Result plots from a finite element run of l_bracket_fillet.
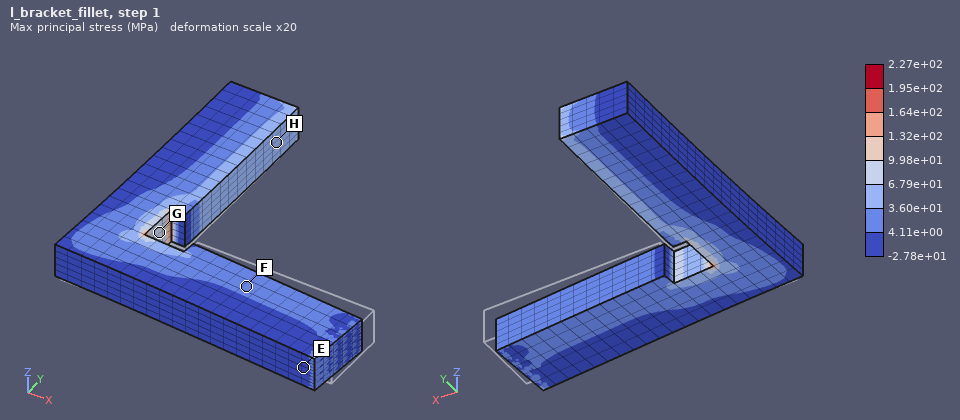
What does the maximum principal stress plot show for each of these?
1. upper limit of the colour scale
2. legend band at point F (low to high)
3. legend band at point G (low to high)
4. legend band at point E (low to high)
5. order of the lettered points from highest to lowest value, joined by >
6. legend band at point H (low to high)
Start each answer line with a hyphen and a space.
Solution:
- 2.27e+02 MPa
- 4.11e+00 to 3.60e+01 MPa
- 6.79e+01 to 9.98e+01 MPa
- -2.78e+01 to 4.11e+00 MPa
- G > H > F > E
- 3.60e+01 to 6.79e+01 MPa
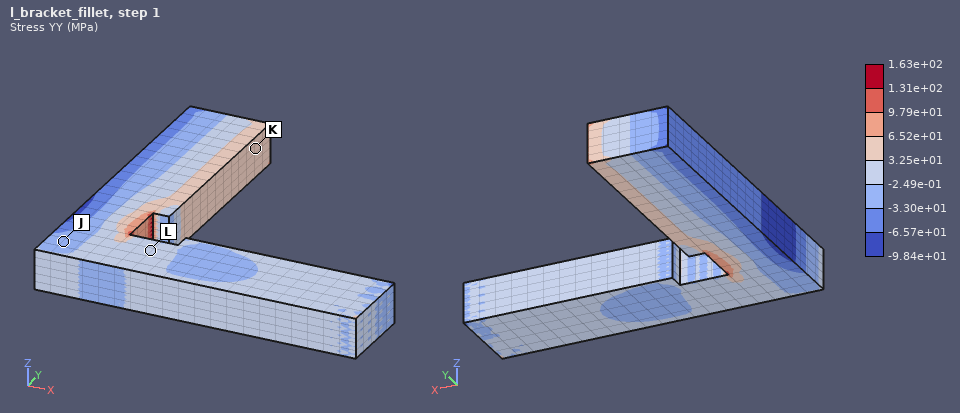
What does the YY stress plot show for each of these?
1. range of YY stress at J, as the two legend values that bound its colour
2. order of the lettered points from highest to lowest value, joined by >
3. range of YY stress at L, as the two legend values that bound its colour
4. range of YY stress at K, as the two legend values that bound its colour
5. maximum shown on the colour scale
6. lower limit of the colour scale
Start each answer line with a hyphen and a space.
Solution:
- -3.30e+01 to -2.49e-01 MPa
- K > L > J
- -2.49e-01 to 3.25e+01 MPa
- 3.25e+01 to 6.52e+01 MPa
- 1.63e+02 MPa
- -9.84e+01 MPa
